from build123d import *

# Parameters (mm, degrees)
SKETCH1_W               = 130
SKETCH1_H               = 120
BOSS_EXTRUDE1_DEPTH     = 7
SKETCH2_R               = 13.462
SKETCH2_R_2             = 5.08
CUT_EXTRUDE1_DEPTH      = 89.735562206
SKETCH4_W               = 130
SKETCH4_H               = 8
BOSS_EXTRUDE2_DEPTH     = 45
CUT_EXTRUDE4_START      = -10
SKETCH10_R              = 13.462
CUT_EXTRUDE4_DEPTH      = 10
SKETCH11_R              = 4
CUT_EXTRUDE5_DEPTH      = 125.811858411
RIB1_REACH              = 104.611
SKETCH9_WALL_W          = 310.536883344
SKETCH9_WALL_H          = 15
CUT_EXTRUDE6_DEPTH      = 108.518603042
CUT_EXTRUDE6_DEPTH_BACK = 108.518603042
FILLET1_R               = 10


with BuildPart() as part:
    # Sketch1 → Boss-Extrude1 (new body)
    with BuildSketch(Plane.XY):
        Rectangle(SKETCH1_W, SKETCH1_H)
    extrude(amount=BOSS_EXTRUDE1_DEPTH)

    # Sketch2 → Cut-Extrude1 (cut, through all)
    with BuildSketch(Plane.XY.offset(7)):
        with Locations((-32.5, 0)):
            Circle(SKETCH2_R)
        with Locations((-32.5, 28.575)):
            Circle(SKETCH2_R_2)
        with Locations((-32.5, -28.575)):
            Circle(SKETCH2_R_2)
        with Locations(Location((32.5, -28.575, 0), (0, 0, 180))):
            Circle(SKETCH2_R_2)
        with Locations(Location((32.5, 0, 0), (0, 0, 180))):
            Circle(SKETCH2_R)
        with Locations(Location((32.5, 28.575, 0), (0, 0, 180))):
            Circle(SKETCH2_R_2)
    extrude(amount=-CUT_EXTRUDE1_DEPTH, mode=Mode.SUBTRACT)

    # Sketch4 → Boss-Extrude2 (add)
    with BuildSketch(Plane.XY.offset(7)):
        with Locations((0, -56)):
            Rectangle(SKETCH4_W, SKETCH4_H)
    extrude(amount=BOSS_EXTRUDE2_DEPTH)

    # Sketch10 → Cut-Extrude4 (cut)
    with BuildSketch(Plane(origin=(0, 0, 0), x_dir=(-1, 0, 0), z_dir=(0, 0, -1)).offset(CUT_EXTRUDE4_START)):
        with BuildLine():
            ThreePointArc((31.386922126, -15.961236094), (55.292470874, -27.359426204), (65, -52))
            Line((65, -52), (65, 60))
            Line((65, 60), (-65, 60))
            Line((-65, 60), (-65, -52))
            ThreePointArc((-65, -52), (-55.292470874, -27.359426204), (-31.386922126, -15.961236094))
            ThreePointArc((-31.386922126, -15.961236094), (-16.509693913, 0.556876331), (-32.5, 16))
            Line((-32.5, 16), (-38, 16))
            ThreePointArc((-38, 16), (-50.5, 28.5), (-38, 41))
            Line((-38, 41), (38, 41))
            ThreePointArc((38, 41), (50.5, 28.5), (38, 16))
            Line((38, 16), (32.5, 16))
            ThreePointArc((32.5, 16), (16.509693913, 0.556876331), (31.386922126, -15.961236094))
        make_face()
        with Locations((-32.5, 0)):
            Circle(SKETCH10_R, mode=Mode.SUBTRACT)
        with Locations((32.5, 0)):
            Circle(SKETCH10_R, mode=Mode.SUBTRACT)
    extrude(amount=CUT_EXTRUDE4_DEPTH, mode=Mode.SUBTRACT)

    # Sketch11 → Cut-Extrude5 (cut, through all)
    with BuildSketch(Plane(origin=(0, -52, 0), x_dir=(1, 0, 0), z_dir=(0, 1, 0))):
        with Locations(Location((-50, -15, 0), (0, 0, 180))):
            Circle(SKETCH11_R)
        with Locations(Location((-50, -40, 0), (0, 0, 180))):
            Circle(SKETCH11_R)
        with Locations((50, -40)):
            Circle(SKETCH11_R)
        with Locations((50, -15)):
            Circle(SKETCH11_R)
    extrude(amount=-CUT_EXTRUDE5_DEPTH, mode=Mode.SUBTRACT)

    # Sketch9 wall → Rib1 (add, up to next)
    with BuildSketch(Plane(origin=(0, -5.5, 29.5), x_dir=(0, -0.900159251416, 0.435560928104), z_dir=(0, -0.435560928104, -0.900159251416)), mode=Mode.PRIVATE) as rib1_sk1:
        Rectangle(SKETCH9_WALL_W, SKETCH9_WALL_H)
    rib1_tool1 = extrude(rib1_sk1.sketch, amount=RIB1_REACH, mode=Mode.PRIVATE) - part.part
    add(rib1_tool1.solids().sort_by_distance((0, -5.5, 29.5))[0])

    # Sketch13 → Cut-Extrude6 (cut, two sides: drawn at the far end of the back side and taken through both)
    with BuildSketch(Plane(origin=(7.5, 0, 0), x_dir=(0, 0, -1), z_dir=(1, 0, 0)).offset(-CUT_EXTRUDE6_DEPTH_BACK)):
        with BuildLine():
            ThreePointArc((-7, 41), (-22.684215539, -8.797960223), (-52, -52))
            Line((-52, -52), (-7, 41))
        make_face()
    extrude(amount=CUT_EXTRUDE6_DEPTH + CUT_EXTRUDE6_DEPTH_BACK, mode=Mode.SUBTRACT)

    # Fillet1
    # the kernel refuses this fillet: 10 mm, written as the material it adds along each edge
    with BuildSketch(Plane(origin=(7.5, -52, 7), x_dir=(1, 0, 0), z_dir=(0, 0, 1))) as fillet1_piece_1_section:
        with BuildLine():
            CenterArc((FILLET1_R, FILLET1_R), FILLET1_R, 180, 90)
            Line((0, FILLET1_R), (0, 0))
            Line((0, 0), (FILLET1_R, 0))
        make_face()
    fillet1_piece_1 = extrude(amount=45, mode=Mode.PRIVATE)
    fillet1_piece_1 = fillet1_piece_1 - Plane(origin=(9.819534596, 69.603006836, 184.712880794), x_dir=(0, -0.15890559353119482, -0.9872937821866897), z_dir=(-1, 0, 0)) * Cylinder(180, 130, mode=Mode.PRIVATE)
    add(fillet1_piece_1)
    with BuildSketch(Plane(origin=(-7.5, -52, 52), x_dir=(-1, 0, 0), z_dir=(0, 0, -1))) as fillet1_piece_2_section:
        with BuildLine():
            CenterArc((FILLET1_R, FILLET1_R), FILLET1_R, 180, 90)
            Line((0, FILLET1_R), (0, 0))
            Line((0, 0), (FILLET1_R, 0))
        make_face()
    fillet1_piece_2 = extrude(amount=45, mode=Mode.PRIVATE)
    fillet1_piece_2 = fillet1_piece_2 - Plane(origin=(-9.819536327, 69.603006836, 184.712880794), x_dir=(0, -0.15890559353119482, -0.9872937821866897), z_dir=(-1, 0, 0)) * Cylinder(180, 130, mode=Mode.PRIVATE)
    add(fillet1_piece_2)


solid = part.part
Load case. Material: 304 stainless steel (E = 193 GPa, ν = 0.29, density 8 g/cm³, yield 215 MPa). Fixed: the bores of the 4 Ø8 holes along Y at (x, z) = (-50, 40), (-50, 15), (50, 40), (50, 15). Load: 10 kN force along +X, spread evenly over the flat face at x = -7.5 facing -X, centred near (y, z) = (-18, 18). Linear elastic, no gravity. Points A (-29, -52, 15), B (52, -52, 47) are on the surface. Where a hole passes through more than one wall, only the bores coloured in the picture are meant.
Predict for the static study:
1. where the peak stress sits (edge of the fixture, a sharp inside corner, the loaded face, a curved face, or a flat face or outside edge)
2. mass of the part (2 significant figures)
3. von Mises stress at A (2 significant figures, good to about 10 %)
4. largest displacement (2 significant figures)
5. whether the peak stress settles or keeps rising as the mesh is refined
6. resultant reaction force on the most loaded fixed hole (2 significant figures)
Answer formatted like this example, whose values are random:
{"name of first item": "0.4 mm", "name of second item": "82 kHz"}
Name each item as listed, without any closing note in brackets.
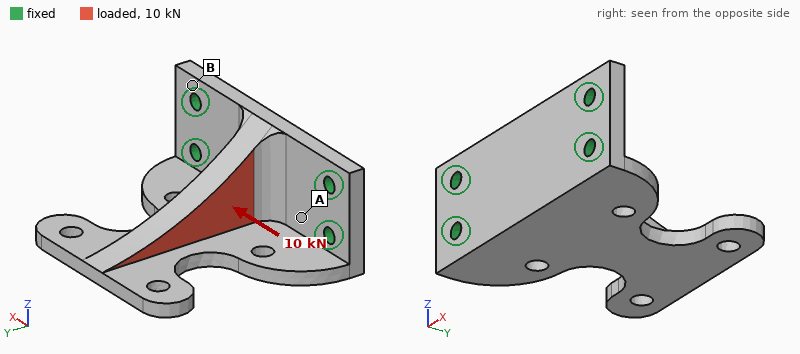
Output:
{"where the peak stress sits": "edge of the fixture", "mass of the part": "1.0 kg", "von Mises stress at A": "26 MPa", "largest displacement": "73 µm", "whether the peak stress settles or keeps rising as the mesh is refined": "keeps rising", "resultant reaction force on the most loaded fixed hole": "5.2 kN"}
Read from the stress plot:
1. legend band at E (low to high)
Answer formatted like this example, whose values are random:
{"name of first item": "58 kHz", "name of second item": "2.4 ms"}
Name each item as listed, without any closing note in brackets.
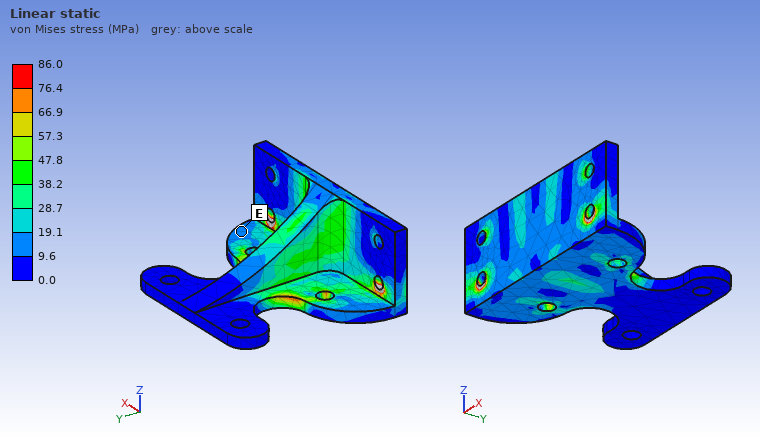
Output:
{"legend band at E": "9.6 to 19.1 MPa"}
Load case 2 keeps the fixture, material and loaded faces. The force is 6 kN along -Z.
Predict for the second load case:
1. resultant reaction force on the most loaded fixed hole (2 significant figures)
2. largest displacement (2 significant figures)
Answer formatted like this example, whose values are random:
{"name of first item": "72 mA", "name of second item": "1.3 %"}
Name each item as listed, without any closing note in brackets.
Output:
{"resultant reaction force on the most loaded fixed hole": "4.6 kN", "largest displacement": "0.24 mm"}
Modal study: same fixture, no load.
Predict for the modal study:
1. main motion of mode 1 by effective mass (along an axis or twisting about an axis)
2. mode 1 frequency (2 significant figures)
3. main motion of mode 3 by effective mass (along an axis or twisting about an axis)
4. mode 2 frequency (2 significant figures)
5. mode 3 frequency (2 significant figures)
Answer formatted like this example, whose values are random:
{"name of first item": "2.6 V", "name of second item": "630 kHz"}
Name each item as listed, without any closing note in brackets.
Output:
{"main motion of mode 1 by effective mass": "along Z", "mode 1 frequency": "1200 Hz", "main motion of mode 3 by effective mass": "along X", "mode 2 frequency": "2000 Hz", "mode 3 frequency": "2900 Hz"}
